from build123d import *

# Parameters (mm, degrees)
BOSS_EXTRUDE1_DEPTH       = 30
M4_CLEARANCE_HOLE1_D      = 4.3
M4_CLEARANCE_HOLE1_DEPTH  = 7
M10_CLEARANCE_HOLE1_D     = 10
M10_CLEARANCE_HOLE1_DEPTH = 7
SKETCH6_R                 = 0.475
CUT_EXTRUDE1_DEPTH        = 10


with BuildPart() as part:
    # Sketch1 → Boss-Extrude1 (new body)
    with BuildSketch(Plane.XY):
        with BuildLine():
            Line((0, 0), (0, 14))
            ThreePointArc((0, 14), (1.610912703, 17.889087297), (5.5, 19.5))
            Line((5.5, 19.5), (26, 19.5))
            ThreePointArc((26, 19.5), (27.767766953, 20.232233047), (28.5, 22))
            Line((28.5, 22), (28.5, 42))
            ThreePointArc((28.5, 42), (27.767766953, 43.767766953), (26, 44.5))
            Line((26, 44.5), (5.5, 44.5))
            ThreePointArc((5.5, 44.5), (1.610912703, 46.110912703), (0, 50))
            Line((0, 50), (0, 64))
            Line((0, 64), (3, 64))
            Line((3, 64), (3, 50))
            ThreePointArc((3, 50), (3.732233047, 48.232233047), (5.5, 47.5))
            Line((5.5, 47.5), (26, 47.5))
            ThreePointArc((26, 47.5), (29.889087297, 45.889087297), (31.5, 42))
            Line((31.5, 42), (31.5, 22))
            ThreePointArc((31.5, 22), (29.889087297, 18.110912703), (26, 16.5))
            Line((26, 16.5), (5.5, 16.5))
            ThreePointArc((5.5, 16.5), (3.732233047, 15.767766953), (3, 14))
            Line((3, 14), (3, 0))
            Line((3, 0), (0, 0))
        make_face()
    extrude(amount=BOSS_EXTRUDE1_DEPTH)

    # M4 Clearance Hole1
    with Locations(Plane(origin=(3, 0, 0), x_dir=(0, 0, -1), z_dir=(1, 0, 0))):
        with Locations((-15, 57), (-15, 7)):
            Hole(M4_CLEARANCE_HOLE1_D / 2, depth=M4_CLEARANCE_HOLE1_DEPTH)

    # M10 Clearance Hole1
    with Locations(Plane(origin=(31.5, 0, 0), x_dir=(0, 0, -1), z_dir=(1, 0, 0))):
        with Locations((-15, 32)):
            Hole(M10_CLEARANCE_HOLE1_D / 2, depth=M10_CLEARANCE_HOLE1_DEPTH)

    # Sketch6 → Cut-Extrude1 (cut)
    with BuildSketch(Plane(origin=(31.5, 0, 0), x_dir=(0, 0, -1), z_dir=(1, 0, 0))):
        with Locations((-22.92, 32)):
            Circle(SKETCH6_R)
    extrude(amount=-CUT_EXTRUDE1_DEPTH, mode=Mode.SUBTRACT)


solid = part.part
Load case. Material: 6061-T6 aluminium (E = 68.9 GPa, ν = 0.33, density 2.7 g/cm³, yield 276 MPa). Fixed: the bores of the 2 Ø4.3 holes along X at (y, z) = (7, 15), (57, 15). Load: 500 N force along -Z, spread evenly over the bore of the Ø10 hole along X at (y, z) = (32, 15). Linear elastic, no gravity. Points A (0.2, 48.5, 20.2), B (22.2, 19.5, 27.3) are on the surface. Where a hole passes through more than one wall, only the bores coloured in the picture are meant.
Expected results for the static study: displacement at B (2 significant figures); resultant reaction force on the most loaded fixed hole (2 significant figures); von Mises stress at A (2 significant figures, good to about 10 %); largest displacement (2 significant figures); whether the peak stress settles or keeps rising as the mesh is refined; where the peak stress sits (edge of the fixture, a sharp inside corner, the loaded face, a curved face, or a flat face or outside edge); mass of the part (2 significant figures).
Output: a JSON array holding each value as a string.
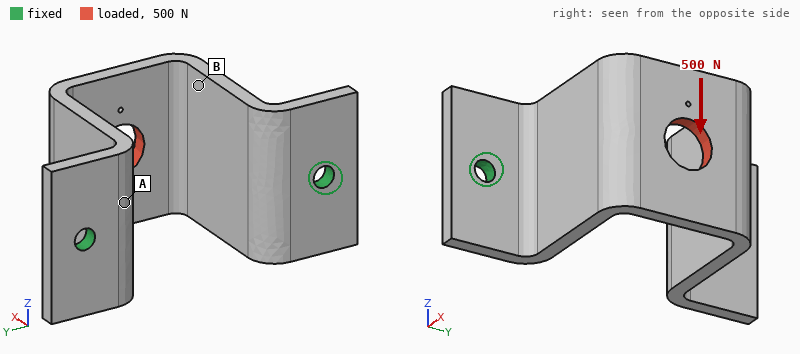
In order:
["0.24 mm", "250 N", "55 MPa", "0.33 mm", "keeps rising", "edge of the fixture", "27 g"]
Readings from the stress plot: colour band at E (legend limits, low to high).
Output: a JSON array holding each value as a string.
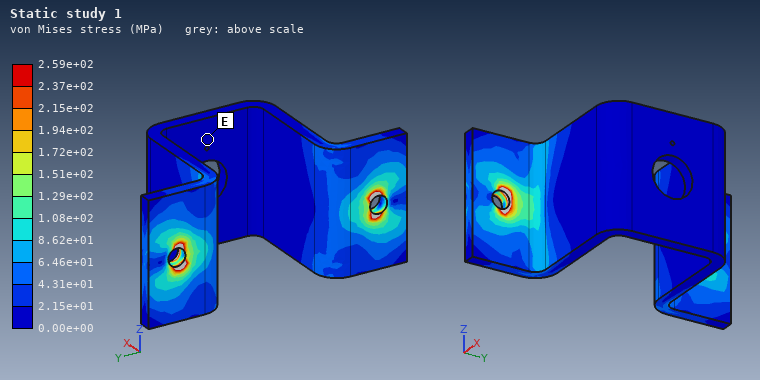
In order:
["0.00e+00 to 2.15e+01 MPa"]
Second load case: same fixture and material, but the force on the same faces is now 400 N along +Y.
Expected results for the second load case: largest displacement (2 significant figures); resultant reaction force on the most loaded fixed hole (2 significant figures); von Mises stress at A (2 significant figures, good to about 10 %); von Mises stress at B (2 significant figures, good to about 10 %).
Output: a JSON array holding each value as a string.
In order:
["0.13 mm", "300 N", "31 MPa", "34 MPa"]
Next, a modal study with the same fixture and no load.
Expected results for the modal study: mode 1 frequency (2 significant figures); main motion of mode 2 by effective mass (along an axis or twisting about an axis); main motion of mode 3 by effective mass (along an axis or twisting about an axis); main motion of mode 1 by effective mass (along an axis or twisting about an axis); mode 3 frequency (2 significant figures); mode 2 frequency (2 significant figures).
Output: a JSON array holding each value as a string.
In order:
["1900 Hz", "along Y", "twisting about X", "along Z", "3800 Hz", "2700 Hz"]
